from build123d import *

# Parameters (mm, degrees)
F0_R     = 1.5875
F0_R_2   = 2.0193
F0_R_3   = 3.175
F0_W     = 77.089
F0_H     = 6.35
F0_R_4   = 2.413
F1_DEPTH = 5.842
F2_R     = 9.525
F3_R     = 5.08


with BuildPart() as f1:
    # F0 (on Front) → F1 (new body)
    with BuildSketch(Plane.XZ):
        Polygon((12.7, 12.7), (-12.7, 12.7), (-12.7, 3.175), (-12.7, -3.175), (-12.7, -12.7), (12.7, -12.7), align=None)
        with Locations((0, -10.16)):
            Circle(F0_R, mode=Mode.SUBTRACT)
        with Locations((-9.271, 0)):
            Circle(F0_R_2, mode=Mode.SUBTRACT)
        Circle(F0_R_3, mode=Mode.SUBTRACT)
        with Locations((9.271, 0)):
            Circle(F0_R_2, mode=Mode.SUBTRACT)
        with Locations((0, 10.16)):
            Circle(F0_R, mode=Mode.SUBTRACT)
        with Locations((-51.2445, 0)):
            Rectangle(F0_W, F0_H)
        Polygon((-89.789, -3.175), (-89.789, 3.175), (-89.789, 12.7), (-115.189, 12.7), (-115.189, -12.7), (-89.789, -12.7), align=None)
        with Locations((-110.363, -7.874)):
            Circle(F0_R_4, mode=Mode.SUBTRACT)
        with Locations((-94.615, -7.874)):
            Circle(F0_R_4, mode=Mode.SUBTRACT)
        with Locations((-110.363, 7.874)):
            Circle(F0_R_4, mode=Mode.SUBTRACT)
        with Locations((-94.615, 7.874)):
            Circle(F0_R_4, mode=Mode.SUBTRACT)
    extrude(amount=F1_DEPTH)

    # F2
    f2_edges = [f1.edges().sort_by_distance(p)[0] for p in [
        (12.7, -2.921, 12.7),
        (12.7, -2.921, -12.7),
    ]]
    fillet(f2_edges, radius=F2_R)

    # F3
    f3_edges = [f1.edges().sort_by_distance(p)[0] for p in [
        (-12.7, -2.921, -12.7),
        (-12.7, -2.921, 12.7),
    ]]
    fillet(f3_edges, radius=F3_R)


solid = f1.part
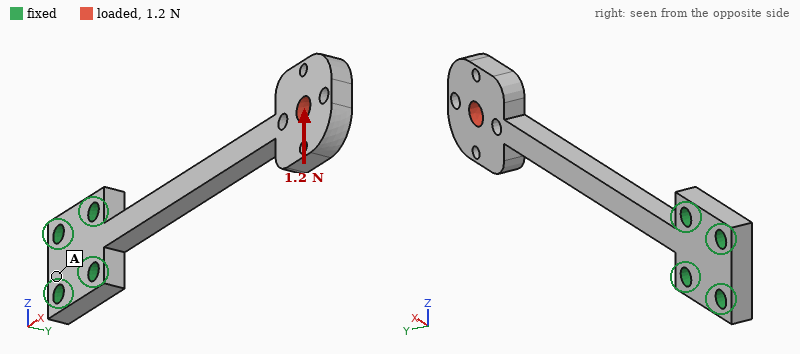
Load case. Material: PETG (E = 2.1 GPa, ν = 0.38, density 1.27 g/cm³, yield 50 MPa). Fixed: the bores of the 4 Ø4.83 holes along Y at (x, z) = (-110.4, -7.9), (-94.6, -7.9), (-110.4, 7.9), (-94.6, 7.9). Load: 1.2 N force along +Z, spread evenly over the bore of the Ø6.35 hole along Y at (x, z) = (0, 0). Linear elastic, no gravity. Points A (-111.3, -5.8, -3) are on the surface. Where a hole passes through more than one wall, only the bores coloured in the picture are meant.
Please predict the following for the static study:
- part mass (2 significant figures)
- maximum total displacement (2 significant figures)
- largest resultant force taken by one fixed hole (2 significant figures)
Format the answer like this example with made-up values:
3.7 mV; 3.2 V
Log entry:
12 g; 1.4 mm; 8.6 N
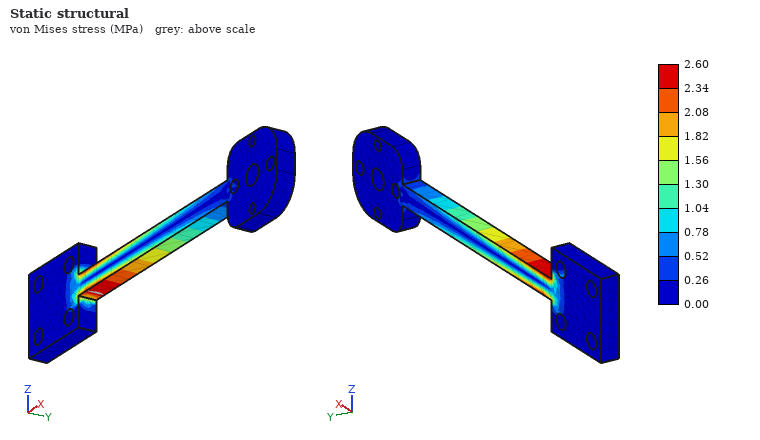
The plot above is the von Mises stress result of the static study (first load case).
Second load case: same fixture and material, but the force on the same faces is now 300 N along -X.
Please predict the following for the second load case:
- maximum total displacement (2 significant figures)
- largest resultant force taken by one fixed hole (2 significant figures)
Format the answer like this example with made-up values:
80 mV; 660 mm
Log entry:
0.37 mm; 130 N
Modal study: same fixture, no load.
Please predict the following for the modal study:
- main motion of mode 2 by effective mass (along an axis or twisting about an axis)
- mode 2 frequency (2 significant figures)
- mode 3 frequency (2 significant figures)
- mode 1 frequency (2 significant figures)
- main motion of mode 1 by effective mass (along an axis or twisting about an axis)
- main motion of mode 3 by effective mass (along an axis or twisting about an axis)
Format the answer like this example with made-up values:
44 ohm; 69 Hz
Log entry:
along Z; 76 Hz; 460 Hz; 68 Hz; along Y; twisting about X
